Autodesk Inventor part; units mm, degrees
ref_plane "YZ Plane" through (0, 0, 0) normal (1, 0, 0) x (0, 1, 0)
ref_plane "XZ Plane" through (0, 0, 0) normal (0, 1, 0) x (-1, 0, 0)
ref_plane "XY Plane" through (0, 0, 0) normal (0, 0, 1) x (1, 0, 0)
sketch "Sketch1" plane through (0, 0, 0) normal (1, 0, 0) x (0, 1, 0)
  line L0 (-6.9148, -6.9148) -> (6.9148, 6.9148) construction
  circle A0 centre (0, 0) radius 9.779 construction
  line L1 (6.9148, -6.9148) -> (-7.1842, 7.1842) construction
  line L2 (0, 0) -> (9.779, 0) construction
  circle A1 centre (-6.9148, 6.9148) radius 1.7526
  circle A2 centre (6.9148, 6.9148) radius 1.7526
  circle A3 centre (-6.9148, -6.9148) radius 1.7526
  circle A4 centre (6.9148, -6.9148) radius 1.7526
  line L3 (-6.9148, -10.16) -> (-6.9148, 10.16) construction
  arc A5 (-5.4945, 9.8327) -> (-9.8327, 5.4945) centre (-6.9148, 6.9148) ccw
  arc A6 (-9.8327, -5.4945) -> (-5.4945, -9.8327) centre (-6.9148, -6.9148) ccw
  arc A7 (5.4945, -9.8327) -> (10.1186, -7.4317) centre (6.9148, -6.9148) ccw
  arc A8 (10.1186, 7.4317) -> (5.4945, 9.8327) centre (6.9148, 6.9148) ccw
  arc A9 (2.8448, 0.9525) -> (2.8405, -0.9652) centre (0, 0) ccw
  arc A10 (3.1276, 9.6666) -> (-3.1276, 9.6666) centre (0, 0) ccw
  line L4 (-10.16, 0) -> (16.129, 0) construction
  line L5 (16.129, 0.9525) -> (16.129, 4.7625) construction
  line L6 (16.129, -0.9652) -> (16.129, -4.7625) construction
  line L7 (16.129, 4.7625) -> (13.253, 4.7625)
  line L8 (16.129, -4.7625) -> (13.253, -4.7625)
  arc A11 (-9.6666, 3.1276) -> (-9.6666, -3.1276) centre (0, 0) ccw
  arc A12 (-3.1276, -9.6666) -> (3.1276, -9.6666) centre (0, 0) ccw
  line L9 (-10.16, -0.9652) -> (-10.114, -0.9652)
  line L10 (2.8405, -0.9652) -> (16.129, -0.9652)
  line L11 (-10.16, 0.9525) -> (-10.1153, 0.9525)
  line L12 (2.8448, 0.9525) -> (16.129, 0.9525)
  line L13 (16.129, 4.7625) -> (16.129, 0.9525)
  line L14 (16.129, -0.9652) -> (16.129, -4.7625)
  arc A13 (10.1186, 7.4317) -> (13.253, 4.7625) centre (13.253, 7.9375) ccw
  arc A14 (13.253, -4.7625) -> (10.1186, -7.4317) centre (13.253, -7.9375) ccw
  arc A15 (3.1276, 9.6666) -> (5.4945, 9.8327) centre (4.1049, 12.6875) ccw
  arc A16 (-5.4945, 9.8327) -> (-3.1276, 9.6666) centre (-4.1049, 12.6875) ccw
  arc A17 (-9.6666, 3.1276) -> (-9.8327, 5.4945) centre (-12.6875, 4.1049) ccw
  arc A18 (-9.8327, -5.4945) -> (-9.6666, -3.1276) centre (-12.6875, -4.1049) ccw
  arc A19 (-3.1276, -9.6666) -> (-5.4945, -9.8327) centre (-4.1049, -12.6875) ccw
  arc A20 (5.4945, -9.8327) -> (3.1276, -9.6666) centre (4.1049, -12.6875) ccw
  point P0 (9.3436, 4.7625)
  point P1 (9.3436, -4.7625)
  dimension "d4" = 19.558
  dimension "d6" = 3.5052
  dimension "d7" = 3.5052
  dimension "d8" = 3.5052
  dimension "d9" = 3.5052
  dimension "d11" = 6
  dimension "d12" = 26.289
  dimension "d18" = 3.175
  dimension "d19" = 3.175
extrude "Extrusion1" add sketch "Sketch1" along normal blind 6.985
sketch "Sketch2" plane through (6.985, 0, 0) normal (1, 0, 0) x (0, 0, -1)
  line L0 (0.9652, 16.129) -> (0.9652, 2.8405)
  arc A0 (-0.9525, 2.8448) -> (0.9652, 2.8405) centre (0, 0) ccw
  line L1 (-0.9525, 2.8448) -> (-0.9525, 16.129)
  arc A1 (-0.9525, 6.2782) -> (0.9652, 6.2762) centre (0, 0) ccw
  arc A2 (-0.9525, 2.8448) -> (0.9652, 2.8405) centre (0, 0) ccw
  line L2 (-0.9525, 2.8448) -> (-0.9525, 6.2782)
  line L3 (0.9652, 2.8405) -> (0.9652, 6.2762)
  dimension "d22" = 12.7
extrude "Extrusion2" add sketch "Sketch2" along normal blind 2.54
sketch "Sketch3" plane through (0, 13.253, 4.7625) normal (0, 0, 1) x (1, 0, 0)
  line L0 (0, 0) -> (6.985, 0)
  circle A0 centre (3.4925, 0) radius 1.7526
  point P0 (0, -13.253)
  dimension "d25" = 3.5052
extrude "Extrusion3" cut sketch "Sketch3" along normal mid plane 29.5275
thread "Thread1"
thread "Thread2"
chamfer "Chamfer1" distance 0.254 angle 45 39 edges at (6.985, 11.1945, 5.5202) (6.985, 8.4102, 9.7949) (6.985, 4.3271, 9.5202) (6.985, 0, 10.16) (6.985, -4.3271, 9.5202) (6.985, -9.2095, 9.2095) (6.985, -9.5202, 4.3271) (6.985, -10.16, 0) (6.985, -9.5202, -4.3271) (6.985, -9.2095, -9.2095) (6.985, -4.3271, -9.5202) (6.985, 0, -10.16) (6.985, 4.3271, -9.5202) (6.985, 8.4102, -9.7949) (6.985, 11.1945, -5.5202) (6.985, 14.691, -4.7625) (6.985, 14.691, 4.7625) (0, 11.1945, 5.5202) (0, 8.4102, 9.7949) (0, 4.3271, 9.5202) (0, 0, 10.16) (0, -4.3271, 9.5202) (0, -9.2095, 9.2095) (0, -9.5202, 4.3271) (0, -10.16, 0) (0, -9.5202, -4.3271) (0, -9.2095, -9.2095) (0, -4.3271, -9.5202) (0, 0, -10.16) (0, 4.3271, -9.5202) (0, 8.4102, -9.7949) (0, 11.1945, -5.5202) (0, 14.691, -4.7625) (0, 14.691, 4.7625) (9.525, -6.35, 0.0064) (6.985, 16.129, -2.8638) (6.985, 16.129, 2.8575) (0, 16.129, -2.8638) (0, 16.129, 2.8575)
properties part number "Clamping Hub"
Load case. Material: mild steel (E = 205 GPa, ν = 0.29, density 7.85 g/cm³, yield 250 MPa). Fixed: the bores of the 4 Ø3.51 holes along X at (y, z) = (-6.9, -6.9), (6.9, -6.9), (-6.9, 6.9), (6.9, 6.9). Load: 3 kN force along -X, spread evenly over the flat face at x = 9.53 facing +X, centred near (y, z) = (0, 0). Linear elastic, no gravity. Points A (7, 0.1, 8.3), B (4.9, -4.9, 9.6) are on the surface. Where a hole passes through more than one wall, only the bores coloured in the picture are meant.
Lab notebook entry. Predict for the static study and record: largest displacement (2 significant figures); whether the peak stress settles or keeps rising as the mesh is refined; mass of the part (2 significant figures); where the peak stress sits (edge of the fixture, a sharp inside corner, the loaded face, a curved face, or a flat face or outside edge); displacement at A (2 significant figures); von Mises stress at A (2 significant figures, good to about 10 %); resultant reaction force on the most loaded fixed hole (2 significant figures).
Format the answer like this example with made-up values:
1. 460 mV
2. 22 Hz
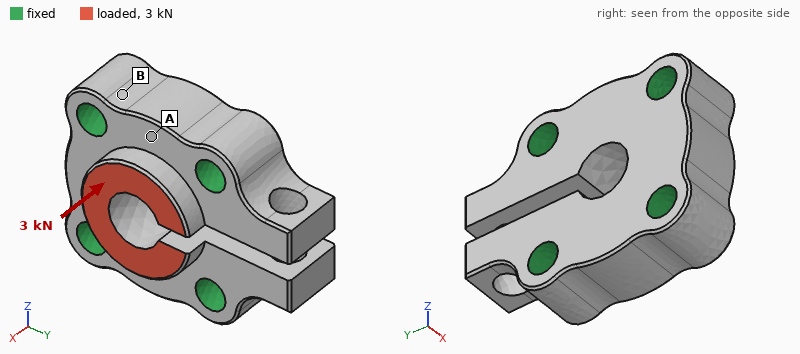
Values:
1. 2.5 µm
2. keeps rising
3. 21 g
4. edge of the fixture
5. 0.50 µm
6. 13 MPa
7. 810 N
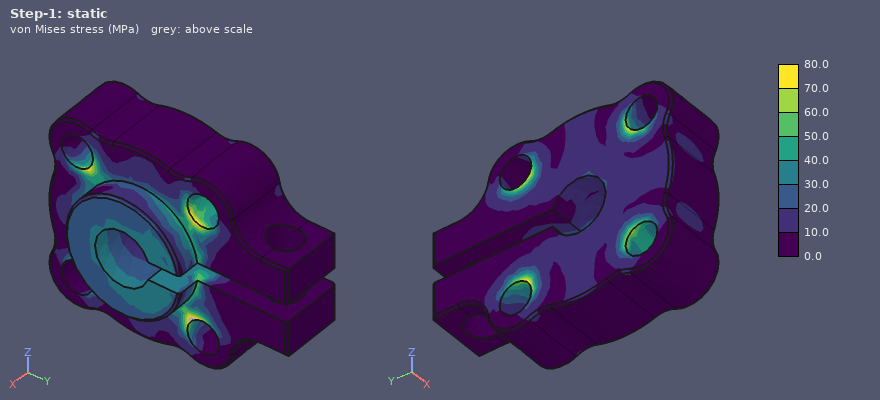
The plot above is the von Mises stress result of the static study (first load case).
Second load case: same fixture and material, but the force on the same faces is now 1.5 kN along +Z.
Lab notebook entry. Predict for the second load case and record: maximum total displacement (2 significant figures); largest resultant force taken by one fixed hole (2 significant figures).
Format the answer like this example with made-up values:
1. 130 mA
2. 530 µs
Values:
1. 3.6 µm
2. 590 N
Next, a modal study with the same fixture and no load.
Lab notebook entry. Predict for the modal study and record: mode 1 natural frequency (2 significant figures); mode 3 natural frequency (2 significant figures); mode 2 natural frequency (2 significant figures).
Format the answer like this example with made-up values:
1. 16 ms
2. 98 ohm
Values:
1. 51 kHz
2. 52 kHz
3. 51 kHz
